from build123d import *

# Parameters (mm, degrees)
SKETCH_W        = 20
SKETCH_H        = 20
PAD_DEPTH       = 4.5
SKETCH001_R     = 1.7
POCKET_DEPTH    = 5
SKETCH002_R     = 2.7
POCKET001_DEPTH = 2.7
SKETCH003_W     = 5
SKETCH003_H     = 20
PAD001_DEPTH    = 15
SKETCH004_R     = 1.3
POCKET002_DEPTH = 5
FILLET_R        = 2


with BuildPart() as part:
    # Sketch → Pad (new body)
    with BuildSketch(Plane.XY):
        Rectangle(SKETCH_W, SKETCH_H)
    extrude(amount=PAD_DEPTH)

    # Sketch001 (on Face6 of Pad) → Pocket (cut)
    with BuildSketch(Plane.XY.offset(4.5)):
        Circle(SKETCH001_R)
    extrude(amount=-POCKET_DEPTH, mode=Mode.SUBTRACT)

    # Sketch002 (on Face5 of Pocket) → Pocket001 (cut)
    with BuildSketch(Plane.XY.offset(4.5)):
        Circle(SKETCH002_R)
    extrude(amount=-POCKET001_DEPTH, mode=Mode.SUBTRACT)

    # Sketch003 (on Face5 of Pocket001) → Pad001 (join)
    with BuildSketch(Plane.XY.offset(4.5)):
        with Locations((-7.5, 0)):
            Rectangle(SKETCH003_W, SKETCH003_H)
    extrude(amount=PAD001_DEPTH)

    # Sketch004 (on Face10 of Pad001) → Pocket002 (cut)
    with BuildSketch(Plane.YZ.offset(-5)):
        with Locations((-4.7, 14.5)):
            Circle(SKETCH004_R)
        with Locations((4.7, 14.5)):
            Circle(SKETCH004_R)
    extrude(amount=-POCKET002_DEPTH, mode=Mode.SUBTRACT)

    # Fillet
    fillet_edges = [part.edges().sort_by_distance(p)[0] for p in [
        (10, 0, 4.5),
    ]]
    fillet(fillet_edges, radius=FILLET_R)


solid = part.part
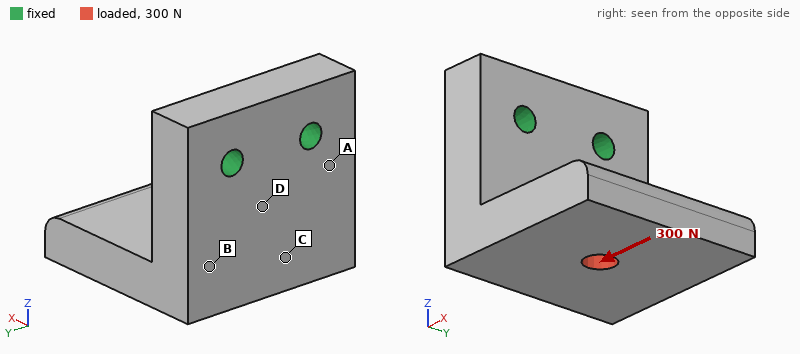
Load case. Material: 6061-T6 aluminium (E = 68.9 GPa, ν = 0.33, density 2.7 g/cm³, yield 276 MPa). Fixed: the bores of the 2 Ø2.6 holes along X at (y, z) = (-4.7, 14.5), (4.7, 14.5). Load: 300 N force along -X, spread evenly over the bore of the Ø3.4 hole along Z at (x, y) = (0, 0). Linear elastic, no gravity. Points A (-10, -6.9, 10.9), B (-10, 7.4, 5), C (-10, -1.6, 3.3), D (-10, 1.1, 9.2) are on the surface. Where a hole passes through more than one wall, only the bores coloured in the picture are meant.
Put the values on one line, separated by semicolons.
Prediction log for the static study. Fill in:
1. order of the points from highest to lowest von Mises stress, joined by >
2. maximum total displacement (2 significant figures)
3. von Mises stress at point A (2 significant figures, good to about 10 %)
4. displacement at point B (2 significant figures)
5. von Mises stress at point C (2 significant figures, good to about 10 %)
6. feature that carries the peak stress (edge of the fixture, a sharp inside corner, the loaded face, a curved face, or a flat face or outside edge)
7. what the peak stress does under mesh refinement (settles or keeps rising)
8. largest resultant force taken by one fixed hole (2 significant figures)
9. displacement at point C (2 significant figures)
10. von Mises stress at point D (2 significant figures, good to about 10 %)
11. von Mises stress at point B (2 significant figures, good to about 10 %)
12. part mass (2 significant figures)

A > D > B > C; 43 µm; 33 MPa; 12 µm; 7.6 MPa; edge of the fixture; keeps rising; 150 N; 15 µm; 26 MPa; 13 MPa; 8.5 g
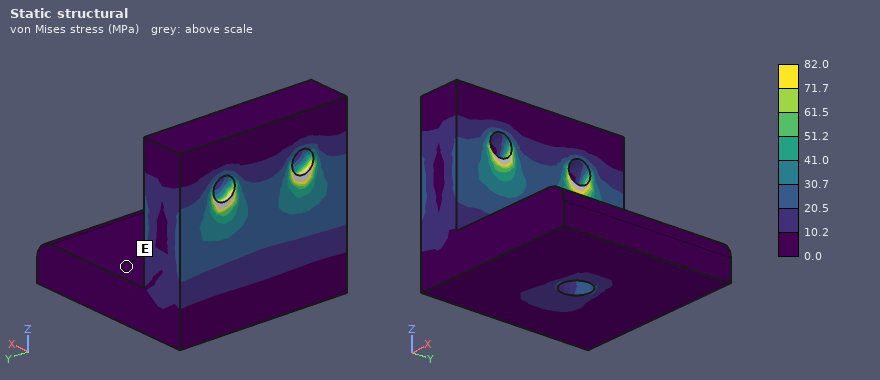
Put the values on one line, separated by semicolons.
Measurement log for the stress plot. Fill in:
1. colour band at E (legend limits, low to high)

0.0 to 10.2 MPa
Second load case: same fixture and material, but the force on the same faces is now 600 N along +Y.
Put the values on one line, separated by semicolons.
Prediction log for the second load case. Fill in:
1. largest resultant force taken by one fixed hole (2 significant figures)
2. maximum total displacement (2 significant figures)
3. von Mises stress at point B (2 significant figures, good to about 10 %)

820 N; 40 µm; 18 MPa
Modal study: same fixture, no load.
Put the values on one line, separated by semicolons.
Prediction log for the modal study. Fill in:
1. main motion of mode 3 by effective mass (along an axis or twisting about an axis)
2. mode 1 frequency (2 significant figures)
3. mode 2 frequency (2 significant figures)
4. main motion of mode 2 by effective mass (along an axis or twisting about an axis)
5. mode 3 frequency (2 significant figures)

along X; 6400 Hz; 9900 Hz; along Y; 16 kHz
